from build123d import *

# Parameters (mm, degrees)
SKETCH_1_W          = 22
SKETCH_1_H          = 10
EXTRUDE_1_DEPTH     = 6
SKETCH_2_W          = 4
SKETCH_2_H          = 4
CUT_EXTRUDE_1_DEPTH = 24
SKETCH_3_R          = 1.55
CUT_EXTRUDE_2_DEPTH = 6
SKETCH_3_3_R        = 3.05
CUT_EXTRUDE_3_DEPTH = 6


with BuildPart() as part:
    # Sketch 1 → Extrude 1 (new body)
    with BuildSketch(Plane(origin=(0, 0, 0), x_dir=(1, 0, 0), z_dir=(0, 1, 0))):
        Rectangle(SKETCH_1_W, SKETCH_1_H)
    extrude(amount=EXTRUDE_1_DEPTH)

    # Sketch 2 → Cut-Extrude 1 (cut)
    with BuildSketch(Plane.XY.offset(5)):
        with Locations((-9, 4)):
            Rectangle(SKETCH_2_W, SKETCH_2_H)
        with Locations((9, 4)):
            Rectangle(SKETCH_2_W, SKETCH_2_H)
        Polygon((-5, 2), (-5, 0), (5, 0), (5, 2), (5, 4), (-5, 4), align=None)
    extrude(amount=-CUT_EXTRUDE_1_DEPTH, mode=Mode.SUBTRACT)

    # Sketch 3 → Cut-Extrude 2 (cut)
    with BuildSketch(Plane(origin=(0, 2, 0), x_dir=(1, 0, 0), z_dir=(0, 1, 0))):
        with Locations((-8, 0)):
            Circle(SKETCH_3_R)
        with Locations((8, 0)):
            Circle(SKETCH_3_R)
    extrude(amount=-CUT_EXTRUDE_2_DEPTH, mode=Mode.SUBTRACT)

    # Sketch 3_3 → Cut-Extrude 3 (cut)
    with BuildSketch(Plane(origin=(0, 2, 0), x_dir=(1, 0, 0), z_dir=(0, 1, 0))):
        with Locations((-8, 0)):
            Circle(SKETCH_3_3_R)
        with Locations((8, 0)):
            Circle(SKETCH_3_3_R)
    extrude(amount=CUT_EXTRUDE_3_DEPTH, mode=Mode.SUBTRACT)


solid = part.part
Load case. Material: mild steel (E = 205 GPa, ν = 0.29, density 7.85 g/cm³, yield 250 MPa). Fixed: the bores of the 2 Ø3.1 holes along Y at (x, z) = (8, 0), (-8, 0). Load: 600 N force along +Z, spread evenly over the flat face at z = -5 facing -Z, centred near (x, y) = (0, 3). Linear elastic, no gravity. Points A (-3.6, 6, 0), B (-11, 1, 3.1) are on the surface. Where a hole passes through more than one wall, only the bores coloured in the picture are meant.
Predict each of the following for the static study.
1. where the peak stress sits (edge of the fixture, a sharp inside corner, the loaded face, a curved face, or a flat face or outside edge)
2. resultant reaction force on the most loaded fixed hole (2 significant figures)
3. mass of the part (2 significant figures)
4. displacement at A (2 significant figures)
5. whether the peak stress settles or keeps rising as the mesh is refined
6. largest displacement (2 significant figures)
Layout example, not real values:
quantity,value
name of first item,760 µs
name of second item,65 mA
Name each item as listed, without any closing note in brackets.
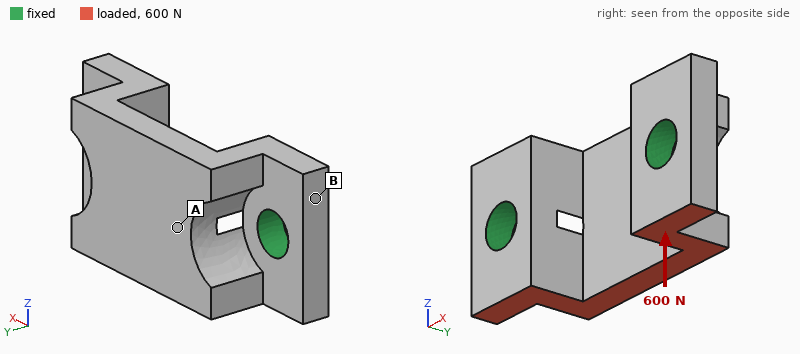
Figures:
quantity,value
where the peak stress sits,a sharp inside corner
resultant reaction force on the most loaded fixed hole,300 N
mass of the part,3.9 g
displacement at A,4.6 µm
whether the peak stress settles or keeps rising as the mesh is refined,keeps rising
largest displacement,6.0 µm
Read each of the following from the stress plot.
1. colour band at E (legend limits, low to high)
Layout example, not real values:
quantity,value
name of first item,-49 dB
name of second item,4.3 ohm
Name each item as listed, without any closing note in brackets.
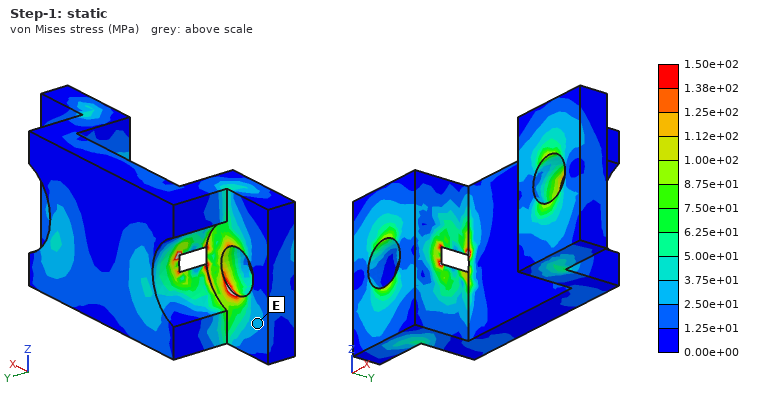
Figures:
quantity,value
colour band at E,2.50e+01 to 3.75e+01 MPa
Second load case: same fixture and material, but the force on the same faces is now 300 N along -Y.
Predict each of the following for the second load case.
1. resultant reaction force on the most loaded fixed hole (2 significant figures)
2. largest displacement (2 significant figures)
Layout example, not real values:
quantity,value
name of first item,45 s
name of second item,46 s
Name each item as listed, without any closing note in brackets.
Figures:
quantity,value
resultant reaction force on the most loaded fixed hole,150 N
largest displacement,6.2 µm
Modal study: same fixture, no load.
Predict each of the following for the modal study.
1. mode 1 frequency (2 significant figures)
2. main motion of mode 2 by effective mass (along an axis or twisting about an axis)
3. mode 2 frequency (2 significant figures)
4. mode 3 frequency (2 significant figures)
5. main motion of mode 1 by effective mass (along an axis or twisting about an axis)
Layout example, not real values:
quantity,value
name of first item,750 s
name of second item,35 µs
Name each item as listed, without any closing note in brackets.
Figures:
quantity,value
mode 1 frequency,28 kHz
main motion of mode 2 by effective mass,along X
mode 2 frequency,35 kHz
mode 3 frequency,43 kHz
main motion of mode 1 by effective mass,along Z
